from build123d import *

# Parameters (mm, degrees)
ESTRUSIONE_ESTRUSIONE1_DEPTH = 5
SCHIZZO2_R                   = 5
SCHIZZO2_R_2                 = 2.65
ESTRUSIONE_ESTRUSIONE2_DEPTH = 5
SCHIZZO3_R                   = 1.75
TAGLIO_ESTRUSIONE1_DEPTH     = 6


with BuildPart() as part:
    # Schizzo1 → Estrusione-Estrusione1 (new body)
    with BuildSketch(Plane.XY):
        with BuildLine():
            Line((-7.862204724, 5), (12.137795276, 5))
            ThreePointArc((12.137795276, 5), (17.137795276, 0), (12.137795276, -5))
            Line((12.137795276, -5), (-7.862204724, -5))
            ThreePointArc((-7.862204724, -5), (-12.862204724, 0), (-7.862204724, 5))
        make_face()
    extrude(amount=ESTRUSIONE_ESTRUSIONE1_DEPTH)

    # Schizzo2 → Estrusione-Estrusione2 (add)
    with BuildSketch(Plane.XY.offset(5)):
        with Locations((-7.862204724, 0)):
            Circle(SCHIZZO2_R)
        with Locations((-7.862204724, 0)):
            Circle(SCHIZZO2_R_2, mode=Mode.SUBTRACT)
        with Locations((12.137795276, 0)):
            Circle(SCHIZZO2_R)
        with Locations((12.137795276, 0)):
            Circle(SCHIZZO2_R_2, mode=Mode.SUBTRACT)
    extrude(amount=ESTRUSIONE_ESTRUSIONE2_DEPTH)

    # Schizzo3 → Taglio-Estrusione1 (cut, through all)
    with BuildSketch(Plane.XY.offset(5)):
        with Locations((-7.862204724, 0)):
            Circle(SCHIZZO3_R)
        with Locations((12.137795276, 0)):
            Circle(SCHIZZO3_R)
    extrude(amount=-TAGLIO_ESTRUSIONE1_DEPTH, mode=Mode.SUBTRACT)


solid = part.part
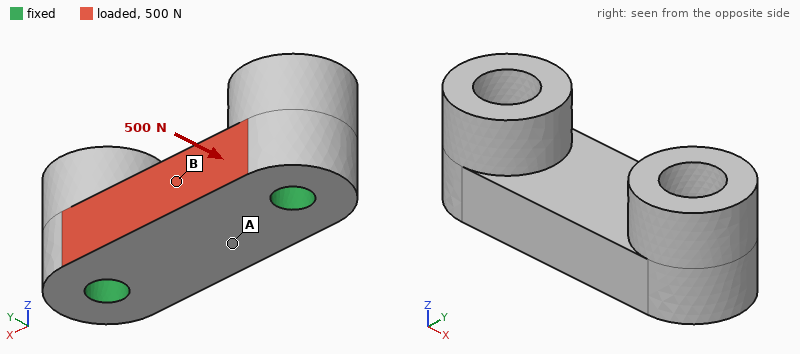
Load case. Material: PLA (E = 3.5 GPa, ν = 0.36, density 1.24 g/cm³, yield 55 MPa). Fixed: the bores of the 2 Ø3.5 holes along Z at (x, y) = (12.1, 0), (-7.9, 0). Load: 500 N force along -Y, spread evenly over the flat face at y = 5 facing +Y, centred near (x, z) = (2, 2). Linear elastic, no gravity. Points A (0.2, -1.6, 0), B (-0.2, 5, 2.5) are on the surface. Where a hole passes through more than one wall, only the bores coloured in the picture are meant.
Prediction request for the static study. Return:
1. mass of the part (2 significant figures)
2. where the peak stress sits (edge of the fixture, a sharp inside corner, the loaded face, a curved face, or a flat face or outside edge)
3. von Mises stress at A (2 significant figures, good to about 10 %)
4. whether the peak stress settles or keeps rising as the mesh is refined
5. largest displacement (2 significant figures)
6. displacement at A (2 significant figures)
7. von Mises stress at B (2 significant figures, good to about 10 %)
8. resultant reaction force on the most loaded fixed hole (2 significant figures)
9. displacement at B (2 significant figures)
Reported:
2.3 g
edge of the fixture
3.4 MPa
keeps rising
34 µm
28 µm
7.9 MPa
250 N
30 µm
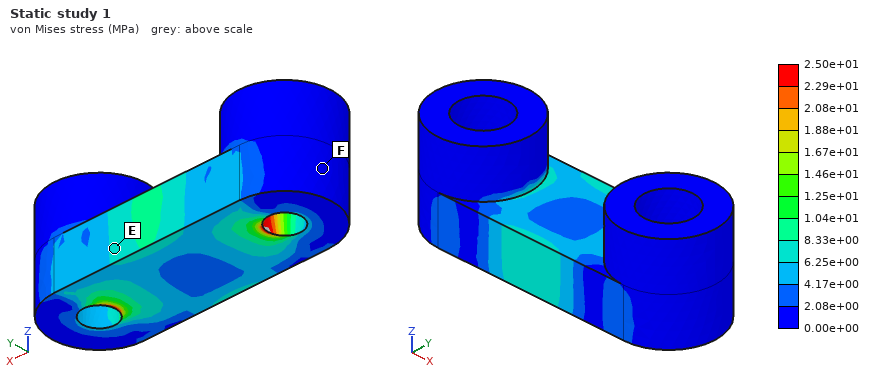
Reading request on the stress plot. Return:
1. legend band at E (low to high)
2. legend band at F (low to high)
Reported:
6.25e+00 to 8.33e+00 MPa
0.00e+00 to 2.08e+00 MPa
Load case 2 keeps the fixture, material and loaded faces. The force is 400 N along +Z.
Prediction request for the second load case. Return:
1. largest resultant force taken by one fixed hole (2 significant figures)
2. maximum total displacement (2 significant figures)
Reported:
200 N
99 µm
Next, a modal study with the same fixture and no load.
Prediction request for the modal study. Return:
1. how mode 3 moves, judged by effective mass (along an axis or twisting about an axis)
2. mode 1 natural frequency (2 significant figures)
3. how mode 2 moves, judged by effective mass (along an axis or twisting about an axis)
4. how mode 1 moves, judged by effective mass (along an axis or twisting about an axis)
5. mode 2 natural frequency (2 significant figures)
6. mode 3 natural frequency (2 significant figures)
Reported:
along Y
16 kHz
along Y
along Z
17 kHz
19 kHz
